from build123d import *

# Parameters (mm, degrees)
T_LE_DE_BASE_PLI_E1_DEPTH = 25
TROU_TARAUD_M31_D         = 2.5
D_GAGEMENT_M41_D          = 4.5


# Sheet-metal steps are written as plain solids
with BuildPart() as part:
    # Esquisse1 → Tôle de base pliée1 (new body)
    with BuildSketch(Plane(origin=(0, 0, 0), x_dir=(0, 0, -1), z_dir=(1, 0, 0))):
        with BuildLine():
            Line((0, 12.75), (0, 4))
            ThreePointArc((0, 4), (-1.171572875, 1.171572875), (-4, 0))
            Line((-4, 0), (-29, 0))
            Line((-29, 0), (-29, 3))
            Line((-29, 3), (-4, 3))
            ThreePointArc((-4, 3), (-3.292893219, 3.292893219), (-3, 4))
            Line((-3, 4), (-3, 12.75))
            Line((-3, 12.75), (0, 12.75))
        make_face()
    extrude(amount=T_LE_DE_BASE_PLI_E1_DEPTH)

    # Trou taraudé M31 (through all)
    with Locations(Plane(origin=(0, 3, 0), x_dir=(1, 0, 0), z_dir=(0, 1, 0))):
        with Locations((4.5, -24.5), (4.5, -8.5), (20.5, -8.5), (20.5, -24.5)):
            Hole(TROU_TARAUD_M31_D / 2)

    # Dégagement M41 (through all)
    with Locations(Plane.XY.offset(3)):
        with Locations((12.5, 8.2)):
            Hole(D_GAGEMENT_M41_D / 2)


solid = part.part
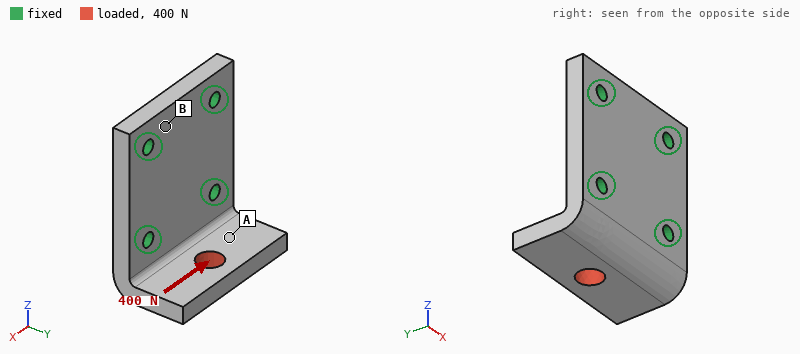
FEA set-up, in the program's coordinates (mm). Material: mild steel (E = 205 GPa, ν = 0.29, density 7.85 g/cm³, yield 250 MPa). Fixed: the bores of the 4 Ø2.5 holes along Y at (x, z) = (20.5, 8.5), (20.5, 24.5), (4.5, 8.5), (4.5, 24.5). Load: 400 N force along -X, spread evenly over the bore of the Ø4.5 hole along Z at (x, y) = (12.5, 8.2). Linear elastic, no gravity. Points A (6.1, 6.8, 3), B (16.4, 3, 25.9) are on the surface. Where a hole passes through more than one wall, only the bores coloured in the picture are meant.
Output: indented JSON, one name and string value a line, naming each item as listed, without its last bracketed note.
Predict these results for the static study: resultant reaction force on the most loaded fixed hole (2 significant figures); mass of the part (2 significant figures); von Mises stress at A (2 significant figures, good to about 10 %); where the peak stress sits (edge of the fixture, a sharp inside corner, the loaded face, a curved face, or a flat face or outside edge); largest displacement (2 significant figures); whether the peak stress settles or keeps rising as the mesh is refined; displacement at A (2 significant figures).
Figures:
{
  "resultant reaction force on the most loaded fixed hole": "290 N",
  "mass of the part": "21 g",
  "von Mises stress at A": "18 MPa",
  "where the peak stress sits": "edge of the fixture",
  "largest displacement": "5.9 µm",
  "whether the peak stress settles or keeps rising as the mesh is refined": "keeps rising",
  "displacement at A": "2.8 µm"
}
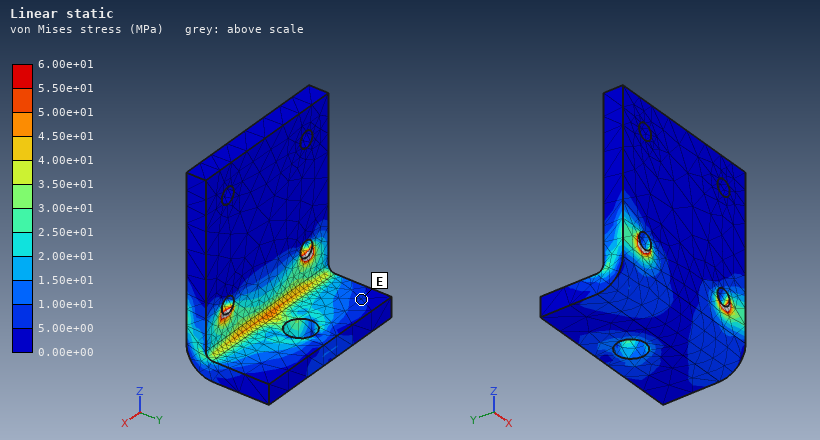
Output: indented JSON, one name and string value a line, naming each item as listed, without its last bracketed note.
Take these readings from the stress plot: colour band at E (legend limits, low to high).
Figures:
{
  "colour band at E": "5.00e+00 to 1.00e+01 MPa"
}
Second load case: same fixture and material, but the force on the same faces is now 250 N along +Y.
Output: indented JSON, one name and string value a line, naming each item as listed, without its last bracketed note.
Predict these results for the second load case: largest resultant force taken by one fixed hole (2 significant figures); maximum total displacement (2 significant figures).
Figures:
{
  "largest resultant force taken by one fixed hole": "140 N",
  "maximum total displacement": "7.9 µm"
}
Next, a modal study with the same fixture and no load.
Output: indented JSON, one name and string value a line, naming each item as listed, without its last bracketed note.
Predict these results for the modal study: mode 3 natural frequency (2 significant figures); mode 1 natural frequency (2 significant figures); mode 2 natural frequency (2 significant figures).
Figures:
{
  "mode 3 natural frequency": "26 kHz",
  "mode 1 natural frequency": "10 kHz",
  "mode 2 natural frequency": "16 kHz"
}
